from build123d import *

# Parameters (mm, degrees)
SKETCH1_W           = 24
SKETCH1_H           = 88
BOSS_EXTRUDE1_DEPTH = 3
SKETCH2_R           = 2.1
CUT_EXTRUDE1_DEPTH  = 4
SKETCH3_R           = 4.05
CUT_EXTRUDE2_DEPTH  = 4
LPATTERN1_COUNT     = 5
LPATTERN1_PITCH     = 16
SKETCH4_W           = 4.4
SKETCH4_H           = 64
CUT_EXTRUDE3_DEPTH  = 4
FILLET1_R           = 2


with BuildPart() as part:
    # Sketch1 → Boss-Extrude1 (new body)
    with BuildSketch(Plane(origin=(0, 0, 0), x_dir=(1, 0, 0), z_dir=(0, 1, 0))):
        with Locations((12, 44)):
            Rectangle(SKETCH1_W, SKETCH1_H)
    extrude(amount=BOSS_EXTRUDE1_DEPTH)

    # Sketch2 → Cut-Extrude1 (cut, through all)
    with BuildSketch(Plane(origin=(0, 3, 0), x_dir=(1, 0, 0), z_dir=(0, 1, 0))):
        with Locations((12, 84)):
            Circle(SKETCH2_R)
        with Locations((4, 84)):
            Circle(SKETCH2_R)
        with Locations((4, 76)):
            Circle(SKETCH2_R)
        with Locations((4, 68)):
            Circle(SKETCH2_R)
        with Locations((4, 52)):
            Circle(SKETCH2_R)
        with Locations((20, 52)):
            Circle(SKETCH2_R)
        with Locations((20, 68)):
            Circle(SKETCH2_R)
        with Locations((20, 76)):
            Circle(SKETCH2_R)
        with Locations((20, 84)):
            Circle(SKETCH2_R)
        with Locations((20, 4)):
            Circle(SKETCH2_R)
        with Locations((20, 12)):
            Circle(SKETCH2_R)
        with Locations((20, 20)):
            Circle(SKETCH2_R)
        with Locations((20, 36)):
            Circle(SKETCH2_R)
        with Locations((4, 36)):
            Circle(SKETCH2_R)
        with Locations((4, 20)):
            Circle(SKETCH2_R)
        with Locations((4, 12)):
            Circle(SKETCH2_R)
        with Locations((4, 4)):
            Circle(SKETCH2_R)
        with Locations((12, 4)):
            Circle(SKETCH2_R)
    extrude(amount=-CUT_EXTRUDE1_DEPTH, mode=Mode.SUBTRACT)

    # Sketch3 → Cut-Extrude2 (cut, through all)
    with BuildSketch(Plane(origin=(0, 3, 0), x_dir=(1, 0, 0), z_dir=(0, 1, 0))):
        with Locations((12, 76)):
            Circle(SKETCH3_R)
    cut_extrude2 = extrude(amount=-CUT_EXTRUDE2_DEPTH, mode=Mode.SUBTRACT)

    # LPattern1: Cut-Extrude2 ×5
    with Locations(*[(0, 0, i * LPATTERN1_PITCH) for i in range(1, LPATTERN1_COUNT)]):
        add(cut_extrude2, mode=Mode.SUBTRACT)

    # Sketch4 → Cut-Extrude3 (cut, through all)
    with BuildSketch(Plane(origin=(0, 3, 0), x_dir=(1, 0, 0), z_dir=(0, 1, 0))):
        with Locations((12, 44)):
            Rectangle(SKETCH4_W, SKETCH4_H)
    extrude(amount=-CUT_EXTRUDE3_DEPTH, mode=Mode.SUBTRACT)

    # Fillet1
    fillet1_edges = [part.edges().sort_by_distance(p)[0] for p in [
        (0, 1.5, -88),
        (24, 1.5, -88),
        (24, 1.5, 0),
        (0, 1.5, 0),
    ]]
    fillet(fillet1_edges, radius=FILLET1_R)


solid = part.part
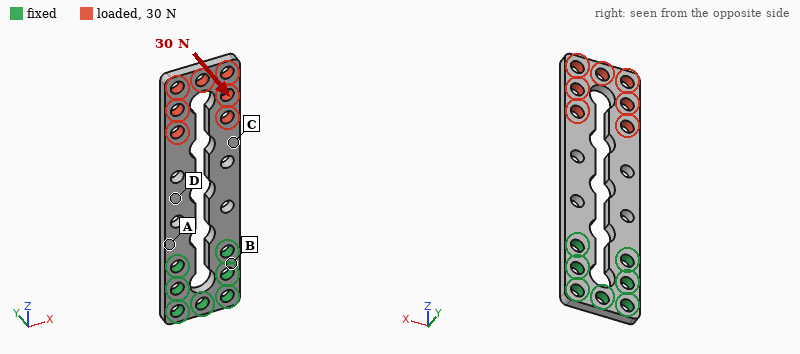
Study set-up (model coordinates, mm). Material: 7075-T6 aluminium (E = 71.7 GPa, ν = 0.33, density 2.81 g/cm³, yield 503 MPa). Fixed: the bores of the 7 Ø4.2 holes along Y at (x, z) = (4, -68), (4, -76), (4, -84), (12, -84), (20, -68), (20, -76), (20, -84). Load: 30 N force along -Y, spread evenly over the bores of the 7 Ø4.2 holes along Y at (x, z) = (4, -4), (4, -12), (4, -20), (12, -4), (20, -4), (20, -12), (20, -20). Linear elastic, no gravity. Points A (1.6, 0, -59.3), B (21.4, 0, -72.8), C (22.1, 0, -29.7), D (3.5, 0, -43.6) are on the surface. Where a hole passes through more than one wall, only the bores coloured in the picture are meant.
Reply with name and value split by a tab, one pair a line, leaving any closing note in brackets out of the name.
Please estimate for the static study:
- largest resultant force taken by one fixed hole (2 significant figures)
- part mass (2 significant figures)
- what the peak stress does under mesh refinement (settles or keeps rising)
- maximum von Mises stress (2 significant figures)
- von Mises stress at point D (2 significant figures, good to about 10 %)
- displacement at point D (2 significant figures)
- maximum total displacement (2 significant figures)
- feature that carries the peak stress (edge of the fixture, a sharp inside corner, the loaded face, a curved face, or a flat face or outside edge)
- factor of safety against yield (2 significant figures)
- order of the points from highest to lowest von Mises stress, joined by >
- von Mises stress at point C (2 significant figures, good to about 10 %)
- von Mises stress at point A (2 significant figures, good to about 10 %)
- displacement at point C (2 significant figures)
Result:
largest resultant force taken by one fixed hole	23 N
part mass	12 g
what the peak stress does under mesh refinement	settles
maximum von Mises stress	120 MPa
von Mises stress at point D	39 MPa
displacement at point D	0.15 mm
maximum total displacement	0.91 mm
feature that carries the peak stress	a curved face
factor of safety against yield	4.0
order of the points from highest to lowest von Mises stress, joined by >	A > D > C > B
von Mises stress at point C	21 MPa
von Mises stress at point A	56 MPa
displacement at point C	0.35 mm
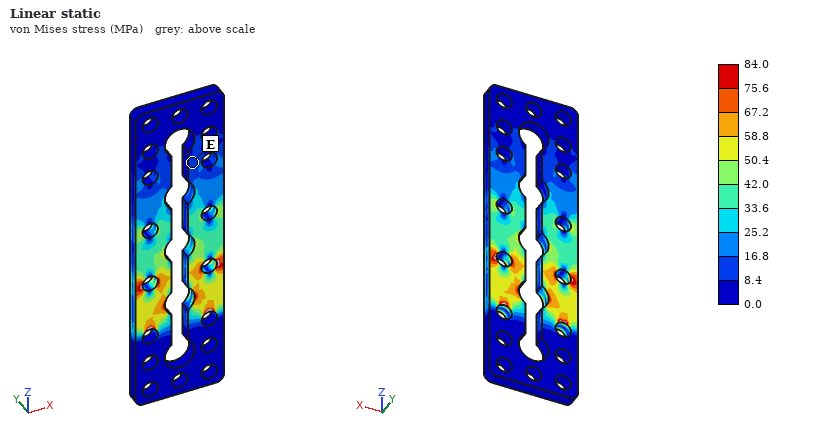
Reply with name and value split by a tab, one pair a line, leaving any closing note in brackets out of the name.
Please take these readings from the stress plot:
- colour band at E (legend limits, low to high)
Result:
colour band at E	8.4 to 16.8 MPa
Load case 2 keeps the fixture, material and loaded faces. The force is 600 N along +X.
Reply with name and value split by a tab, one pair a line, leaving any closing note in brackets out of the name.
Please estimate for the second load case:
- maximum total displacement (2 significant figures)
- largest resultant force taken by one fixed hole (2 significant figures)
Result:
maximum total displacement	0.83 mm
largest resultant force taken by one fixed hole	1.2 kN
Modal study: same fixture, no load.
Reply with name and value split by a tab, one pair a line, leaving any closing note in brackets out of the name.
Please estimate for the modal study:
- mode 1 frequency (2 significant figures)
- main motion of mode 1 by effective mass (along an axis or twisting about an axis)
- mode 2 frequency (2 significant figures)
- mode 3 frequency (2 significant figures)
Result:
mode 1 frequency	530 Hz
main motion of mode 1 by effective mass	along Y
mode 2 frequency	2200 Hz
mode 3 frequency	2300 Hz
